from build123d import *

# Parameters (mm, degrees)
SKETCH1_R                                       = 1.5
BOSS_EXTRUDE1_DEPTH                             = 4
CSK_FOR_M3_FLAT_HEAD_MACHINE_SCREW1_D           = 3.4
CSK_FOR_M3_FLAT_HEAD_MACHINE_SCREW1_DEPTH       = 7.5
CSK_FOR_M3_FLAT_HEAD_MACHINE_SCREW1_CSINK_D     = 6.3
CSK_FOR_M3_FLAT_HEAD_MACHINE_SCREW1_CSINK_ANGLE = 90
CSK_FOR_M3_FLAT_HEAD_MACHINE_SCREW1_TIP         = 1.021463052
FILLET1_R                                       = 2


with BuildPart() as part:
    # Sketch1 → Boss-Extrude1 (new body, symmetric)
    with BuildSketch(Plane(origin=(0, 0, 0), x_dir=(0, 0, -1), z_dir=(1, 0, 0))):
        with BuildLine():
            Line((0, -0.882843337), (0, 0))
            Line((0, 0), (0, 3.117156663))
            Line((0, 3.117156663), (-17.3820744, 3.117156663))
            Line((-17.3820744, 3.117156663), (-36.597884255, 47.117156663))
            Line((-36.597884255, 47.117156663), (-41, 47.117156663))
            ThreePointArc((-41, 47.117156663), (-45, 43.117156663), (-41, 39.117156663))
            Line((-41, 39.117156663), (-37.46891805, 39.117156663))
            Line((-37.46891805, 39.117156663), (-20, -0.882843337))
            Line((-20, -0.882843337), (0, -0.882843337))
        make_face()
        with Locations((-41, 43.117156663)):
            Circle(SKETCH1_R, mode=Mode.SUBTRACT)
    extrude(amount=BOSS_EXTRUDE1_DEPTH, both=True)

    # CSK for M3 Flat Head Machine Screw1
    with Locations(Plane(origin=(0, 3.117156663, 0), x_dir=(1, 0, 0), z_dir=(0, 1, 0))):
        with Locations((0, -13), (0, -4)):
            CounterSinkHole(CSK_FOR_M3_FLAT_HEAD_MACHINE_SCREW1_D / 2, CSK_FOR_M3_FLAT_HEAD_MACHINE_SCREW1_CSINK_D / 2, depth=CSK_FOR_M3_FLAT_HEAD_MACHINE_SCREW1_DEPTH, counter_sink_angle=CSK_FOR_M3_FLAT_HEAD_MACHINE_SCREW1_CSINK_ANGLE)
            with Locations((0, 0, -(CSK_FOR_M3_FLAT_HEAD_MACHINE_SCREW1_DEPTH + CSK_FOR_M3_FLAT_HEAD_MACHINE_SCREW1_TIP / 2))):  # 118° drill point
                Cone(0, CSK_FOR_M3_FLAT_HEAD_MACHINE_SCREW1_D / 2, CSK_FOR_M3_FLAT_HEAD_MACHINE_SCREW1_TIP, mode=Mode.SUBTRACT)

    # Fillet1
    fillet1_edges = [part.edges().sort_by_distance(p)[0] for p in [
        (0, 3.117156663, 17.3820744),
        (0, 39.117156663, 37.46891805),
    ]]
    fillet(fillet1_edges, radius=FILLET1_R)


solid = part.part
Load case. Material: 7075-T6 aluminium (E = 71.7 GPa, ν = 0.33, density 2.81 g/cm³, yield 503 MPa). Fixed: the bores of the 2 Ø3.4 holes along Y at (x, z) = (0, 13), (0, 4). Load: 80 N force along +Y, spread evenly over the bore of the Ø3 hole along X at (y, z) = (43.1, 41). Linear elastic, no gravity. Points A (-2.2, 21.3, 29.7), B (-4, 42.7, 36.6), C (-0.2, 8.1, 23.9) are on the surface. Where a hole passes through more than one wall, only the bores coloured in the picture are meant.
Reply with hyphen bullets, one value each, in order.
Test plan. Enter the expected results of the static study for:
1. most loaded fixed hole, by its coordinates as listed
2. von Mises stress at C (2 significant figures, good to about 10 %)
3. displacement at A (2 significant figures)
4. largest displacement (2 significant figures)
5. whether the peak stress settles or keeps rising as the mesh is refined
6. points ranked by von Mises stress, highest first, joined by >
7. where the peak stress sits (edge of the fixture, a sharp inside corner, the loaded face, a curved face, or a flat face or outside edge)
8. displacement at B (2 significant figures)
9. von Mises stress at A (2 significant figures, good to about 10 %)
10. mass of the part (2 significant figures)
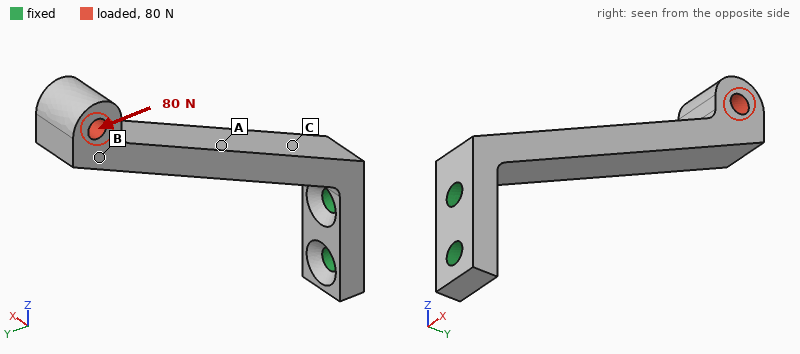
- (0, 13)
- 73 MPa
- 0.23 mm
- 0.74 mm
- keeps rising
- C > A > B
- edge of the fixture
- 0.61 mm
- 52 MPa
- 6.6 g
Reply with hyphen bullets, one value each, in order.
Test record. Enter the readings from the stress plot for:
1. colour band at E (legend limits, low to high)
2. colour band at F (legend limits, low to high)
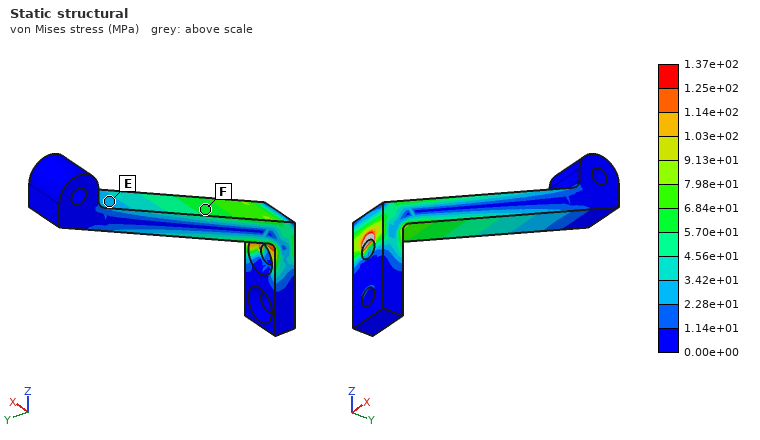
- 2.28e+01 to 3.42e+01 MPa
- 5.70e+01 to 6.84e+01 MPa
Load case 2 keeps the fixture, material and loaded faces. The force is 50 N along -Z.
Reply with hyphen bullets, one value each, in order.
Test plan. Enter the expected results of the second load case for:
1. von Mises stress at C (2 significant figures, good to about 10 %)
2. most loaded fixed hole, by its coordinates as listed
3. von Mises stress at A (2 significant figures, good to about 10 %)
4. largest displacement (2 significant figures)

- 79 MPa
- (0, 4)
- 49 MPa
- 0.78 mm
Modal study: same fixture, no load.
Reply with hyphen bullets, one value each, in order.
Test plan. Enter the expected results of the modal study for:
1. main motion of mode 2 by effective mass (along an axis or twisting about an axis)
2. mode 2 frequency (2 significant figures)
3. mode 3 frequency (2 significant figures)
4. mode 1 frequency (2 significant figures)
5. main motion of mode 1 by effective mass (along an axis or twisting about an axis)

- along X
- 1400 Hz
- 5800 Hz
- 860 Hz
- along Z
